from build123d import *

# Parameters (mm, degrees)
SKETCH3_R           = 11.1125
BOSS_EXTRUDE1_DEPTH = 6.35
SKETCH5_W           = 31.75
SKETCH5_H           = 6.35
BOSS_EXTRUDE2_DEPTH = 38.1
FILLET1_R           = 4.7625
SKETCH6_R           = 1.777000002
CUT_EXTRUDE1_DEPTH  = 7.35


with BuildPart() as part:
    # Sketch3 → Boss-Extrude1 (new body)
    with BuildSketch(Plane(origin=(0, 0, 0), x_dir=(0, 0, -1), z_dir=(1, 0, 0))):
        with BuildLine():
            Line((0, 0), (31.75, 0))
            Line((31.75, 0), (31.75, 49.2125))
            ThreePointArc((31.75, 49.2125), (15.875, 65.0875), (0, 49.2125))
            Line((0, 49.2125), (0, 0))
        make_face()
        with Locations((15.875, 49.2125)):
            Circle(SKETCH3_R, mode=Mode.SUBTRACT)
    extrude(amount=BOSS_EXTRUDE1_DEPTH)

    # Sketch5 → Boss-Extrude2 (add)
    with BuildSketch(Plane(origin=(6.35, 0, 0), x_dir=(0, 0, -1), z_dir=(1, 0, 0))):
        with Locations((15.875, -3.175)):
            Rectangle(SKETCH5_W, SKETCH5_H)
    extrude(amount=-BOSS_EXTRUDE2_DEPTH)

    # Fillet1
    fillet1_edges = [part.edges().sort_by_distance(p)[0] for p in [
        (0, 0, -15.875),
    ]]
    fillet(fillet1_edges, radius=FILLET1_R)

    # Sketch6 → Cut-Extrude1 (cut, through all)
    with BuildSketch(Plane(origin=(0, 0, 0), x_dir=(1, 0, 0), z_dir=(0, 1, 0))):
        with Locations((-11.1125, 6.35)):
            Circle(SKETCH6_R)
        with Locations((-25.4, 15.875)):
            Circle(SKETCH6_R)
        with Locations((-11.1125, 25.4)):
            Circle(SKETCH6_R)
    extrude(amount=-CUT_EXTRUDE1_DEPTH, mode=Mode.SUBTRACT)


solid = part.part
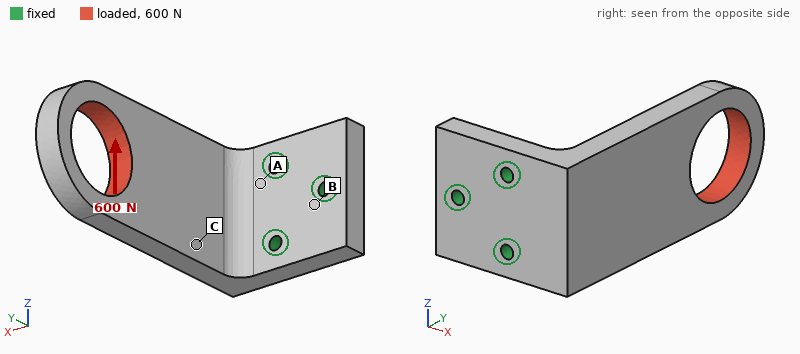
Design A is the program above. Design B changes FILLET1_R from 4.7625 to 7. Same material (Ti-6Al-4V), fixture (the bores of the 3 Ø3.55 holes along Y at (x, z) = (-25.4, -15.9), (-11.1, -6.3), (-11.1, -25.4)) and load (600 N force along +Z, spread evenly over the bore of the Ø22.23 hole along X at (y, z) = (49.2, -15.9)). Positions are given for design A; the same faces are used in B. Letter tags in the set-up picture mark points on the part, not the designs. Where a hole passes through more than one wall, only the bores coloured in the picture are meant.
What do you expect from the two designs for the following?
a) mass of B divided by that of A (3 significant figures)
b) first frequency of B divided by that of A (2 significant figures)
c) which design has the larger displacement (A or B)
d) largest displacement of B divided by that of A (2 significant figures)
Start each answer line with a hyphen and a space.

- 1.01
- 1.1
- A
- 0.90
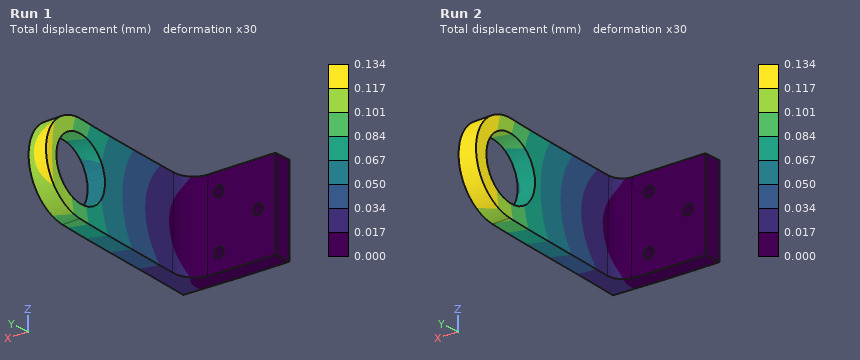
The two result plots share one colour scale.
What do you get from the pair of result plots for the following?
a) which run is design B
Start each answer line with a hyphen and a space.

- Run 1
